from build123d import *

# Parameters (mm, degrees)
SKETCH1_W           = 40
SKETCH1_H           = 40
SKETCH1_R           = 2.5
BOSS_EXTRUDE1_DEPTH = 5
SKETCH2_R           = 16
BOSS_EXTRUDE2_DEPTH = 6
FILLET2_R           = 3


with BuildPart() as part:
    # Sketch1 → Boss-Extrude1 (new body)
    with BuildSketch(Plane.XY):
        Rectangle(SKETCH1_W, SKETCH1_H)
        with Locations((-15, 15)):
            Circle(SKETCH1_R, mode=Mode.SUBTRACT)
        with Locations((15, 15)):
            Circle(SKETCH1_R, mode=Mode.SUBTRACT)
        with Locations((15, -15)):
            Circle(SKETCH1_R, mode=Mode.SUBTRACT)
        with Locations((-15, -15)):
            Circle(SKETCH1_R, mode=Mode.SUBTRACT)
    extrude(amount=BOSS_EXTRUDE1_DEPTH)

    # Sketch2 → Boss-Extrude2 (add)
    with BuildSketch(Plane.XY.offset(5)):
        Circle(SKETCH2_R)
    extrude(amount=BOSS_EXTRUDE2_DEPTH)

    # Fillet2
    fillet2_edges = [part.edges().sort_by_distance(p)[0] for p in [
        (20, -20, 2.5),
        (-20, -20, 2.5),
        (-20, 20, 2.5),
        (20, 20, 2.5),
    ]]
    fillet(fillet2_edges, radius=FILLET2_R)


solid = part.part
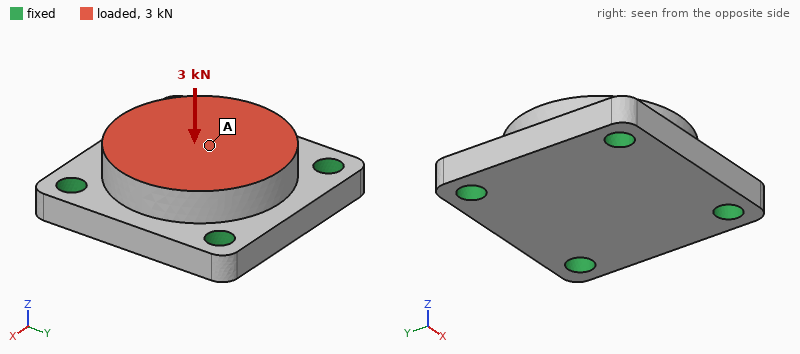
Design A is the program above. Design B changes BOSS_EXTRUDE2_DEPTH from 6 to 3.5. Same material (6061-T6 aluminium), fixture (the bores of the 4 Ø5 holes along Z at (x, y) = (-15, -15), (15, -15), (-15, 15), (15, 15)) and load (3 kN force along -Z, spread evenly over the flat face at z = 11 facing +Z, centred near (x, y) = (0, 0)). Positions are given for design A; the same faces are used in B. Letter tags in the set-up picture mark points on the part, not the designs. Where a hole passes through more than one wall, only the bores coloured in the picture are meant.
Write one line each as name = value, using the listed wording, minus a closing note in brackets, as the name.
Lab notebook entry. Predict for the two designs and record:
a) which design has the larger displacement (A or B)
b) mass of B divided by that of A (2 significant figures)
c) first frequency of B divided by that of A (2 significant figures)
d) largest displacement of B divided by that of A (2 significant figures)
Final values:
which design has the larger displacement = B
mass of B divided by that of A = 0.84
first frequency of B divided by that of A = 1.0
largest displacement of B divided by that of A = 1.3
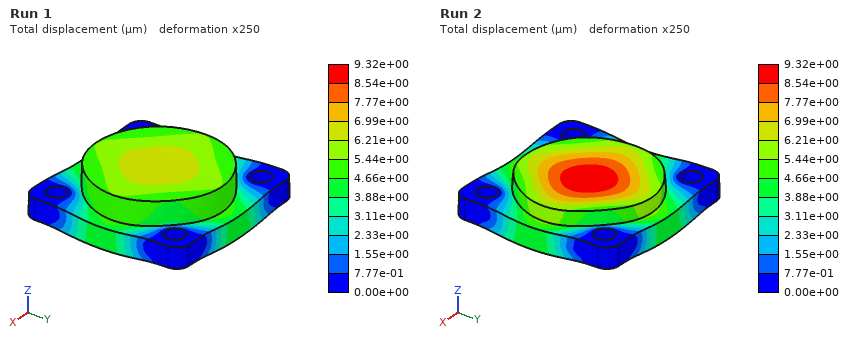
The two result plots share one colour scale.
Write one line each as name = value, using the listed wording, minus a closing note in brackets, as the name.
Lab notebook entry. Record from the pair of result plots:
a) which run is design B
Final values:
which run is design B = Run 2
